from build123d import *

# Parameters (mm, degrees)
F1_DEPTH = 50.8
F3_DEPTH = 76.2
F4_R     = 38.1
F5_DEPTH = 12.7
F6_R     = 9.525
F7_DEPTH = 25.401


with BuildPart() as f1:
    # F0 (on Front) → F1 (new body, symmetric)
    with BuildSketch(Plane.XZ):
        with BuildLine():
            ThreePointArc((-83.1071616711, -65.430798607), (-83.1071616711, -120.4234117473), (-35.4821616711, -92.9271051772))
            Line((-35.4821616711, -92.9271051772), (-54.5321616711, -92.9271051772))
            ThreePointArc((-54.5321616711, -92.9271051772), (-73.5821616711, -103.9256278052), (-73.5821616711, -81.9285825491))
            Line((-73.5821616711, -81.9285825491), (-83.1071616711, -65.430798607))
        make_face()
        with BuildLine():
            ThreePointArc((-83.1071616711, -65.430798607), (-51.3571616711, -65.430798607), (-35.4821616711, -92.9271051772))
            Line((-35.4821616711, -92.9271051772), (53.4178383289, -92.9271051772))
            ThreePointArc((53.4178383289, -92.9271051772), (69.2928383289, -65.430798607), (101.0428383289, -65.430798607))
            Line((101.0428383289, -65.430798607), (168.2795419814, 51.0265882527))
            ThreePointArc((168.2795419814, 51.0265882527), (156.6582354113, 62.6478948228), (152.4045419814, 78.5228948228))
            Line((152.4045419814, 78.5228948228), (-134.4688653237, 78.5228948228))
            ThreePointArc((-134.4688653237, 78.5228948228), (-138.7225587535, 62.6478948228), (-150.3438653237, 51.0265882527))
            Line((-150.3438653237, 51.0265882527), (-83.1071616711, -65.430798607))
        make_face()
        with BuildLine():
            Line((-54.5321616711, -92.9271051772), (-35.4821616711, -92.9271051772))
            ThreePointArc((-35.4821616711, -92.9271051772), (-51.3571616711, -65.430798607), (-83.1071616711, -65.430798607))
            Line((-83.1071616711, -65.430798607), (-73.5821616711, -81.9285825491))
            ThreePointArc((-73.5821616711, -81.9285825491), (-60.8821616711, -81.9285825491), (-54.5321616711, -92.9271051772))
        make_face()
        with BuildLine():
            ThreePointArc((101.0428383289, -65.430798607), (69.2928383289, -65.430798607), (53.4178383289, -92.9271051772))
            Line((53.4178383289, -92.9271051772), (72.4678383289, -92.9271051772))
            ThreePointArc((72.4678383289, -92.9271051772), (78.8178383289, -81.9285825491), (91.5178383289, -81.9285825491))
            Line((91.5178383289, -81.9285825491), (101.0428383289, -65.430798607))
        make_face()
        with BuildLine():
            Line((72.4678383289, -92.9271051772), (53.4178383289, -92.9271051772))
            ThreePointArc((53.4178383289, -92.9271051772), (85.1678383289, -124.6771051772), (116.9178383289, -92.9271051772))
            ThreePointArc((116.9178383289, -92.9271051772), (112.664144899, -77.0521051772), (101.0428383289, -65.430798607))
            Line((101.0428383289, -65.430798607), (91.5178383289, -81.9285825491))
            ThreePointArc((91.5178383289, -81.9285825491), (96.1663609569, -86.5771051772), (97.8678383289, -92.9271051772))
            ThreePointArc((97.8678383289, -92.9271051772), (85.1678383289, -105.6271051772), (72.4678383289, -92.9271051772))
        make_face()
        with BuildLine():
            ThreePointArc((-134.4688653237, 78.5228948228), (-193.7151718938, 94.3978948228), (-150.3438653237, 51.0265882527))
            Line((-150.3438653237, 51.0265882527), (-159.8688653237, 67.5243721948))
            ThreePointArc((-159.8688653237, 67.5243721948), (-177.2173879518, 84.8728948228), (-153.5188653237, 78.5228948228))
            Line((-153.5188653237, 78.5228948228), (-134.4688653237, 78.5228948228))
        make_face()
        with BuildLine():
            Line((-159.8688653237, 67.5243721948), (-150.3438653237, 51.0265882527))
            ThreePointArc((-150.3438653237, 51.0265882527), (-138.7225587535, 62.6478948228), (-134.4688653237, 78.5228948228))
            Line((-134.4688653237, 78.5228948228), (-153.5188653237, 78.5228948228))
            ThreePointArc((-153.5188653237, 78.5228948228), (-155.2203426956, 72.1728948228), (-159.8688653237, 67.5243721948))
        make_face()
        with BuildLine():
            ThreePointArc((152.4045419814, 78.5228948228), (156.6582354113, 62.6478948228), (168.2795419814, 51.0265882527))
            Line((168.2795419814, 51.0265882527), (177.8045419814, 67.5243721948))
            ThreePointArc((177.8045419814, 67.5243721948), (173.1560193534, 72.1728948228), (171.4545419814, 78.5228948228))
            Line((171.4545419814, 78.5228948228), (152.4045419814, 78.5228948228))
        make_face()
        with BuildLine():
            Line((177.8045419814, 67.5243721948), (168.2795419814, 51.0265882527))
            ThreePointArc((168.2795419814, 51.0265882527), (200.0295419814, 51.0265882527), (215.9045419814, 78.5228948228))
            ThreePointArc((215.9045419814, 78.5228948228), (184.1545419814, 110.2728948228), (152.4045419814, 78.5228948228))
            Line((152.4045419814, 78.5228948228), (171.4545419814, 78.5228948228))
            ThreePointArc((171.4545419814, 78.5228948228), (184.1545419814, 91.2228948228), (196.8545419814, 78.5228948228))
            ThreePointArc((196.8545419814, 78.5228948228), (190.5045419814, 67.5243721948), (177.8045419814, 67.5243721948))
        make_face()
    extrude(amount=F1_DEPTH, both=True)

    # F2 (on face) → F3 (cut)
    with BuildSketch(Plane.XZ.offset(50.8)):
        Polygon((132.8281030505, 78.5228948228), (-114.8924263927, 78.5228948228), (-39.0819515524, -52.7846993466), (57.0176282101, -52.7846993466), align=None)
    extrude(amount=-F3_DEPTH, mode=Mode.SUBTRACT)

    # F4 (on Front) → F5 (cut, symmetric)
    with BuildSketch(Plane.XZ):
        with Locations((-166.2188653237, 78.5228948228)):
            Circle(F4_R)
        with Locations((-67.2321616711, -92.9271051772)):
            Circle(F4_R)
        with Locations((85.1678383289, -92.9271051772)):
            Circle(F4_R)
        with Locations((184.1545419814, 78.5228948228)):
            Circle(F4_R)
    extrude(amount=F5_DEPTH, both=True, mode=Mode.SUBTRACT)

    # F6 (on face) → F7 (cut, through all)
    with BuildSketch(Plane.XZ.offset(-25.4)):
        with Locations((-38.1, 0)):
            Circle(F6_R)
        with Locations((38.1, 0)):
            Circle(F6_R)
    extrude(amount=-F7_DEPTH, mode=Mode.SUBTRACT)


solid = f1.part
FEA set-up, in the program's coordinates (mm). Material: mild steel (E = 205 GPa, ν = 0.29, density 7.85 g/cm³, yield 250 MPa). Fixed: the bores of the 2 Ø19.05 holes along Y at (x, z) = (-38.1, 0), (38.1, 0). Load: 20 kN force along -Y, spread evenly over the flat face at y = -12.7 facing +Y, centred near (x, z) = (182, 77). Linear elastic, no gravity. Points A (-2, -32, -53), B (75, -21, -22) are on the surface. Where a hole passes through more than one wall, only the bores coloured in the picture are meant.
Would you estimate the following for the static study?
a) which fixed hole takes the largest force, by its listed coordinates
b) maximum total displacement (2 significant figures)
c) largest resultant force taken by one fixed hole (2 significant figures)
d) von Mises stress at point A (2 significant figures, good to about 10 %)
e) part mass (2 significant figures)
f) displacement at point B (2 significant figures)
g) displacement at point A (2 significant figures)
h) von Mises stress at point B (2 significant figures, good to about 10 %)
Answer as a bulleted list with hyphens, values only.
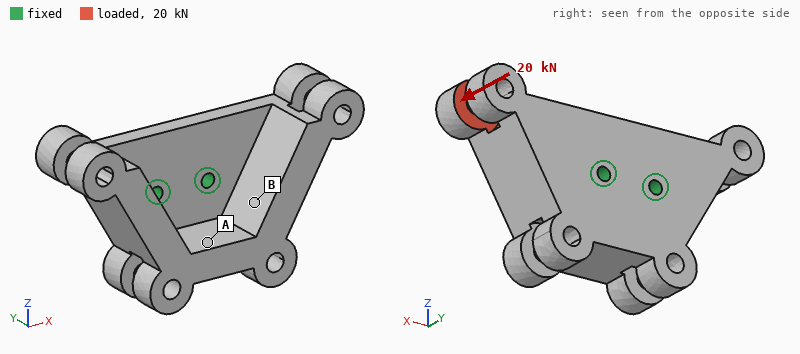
- (38.1, 0)
- 0.36 mm
- 42 kN
- 16 MPa
- 24 kg
- 0.072 mm
- 0.072 mm
- 37 MPa
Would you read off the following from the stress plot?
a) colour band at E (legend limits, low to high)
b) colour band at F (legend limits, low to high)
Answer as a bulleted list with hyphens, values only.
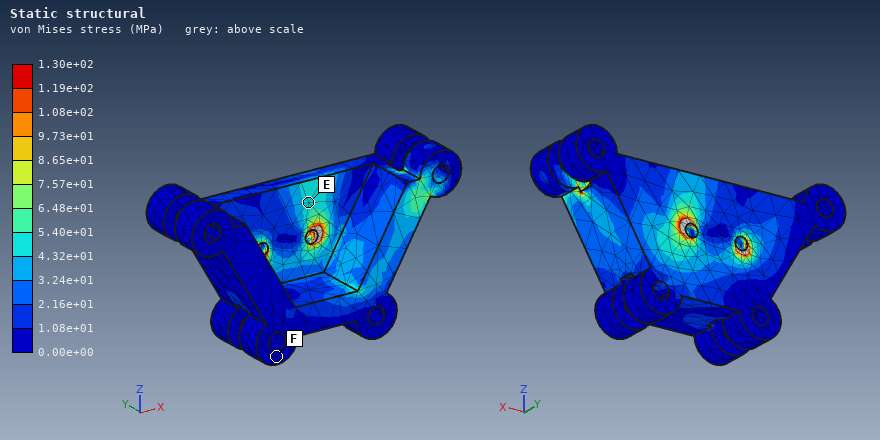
- 4.32e+01 to 5.40e+01 MPa
- 0.00e+00 to 1.08e+01 MPa
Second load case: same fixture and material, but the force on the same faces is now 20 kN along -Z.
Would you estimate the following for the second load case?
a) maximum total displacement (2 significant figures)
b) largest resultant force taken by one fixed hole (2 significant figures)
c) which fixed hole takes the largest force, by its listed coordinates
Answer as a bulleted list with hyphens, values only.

- 0.21 mm
- 50 kN
- (38.1, 0)
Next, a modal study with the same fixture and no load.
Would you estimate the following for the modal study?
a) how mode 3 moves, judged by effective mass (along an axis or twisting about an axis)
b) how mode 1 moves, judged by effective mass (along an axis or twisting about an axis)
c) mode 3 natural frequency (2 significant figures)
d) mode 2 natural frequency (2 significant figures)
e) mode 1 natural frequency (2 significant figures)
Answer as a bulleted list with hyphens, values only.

- twisting about Y
- along Z
- 1200 Hz
- 760 Hz
- 670 Hz
